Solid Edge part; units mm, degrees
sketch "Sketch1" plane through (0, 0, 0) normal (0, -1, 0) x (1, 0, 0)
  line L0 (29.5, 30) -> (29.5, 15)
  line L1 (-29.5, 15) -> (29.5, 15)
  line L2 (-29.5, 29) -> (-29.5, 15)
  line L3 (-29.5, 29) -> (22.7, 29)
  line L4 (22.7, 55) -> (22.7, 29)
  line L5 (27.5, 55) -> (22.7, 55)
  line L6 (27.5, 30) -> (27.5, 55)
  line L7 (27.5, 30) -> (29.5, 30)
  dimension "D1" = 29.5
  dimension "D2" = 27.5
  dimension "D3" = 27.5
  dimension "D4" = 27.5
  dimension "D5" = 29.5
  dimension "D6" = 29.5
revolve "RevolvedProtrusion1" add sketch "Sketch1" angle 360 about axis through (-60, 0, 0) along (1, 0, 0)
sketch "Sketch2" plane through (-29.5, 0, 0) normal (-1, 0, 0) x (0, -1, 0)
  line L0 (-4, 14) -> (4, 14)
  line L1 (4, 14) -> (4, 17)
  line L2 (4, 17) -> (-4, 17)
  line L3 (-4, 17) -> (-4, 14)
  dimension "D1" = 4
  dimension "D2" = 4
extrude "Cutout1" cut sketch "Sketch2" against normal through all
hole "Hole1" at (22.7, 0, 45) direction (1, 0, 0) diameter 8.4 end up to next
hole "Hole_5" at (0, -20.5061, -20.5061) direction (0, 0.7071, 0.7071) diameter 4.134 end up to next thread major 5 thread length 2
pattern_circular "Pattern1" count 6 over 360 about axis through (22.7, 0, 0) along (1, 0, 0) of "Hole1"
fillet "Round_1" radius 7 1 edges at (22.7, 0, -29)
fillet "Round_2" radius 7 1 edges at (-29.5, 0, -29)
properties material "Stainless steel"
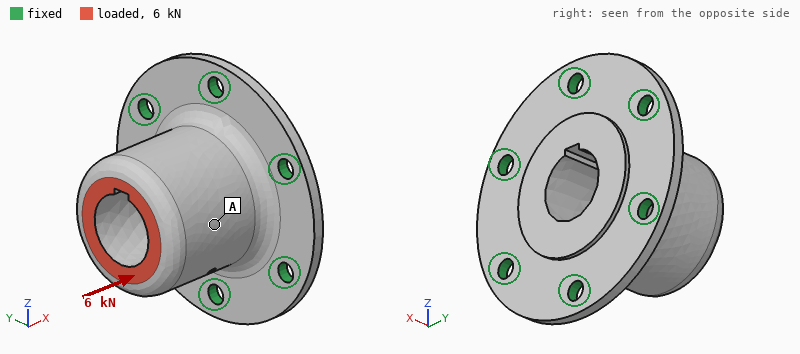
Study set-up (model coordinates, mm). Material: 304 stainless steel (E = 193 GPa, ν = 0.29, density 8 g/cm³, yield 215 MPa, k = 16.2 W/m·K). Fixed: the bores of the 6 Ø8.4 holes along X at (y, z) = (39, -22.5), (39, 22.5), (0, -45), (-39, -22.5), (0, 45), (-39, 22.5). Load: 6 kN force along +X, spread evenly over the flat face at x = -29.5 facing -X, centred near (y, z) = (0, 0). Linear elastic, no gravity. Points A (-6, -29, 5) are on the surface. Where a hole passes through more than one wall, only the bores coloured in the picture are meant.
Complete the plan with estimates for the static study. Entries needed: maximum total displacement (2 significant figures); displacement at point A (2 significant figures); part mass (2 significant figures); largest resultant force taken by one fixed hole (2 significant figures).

7.1 µm
6.4 µm
1.2 kg
1.2 kN
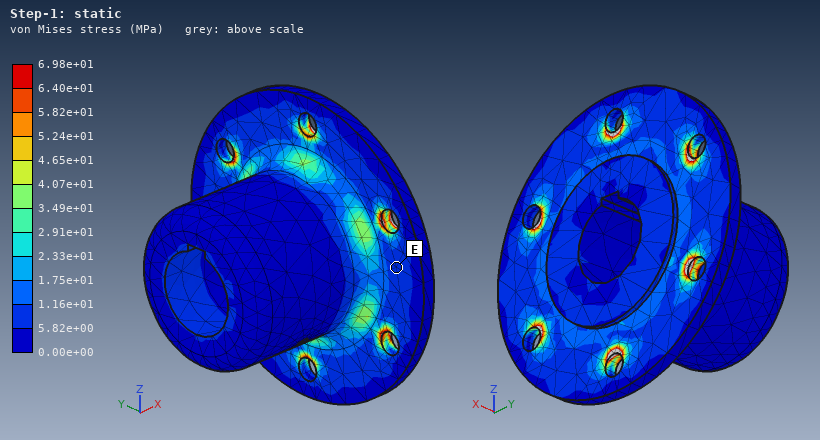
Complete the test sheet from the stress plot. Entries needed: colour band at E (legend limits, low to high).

5.82e+00 to 1.16e+01 MPa
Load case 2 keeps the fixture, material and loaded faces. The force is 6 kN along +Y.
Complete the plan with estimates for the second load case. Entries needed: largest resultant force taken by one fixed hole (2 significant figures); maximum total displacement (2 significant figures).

2.9 kN
32 µm
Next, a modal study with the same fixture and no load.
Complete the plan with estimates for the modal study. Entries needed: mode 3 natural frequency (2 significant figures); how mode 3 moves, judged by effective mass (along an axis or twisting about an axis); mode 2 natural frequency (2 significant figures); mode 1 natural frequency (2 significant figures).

5100 Hz
along X
4000 Hz
4000 Hz
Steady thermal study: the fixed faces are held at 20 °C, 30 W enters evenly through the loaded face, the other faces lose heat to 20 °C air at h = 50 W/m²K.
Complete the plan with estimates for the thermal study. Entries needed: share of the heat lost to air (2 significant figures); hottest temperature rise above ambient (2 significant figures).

73 %
49 K
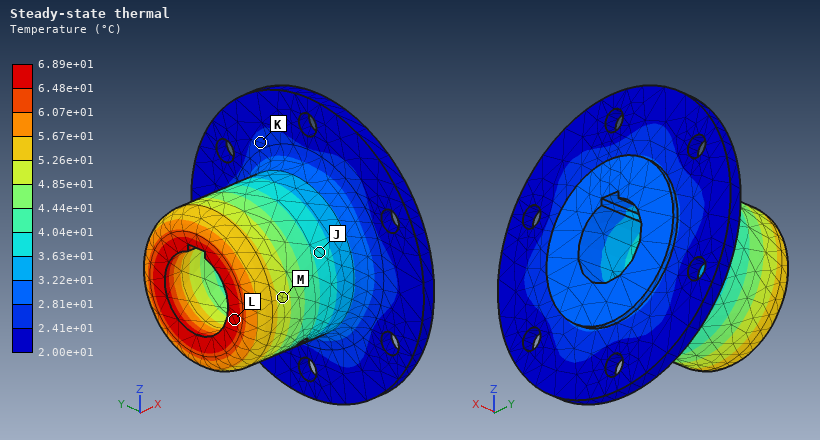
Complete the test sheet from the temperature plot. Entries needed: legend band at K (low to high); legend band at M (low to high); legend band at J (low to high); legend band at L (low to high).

2.41e+01 to 2.81e+01 °C
4.85e+01 to 5.26e+01 °C
3.63e+01 to 4.04e+01 °C
6.48e+01 to 6.89e+01 °C
